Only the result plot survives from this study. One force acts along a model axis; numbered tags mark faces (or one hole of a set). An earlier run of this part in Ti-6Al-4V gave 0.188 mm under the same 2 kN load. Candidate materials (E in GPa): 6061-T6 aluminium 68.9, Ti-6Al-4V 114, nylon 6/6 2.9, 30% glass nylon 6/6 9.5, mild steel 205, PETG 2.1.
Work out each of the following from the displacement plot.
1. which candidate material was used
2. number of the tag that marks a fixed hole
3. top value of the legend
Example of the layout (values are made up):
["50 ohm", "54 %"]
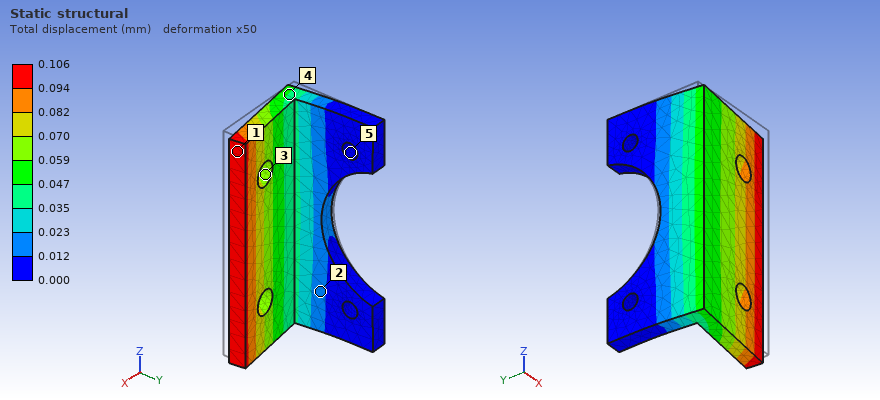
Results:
["mild steel", "5", "0.106 mm"]
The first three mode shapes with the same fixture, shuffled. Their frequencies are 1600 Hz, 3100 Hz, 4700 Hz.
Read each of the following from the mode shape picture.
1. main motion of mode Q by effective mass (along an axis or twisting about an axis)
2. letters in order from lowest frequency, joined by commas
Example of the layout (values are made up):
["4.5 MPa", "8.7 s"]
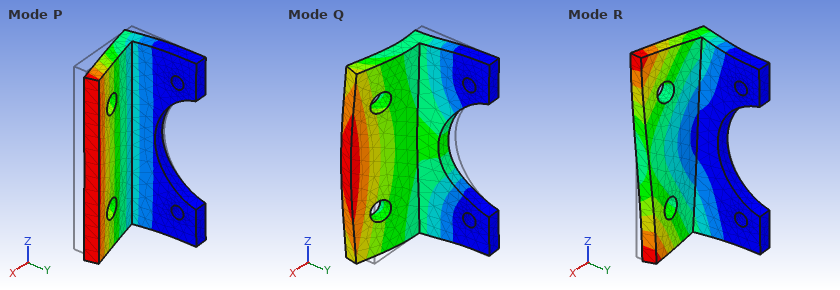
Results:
["along X", "P, R, Q"]
